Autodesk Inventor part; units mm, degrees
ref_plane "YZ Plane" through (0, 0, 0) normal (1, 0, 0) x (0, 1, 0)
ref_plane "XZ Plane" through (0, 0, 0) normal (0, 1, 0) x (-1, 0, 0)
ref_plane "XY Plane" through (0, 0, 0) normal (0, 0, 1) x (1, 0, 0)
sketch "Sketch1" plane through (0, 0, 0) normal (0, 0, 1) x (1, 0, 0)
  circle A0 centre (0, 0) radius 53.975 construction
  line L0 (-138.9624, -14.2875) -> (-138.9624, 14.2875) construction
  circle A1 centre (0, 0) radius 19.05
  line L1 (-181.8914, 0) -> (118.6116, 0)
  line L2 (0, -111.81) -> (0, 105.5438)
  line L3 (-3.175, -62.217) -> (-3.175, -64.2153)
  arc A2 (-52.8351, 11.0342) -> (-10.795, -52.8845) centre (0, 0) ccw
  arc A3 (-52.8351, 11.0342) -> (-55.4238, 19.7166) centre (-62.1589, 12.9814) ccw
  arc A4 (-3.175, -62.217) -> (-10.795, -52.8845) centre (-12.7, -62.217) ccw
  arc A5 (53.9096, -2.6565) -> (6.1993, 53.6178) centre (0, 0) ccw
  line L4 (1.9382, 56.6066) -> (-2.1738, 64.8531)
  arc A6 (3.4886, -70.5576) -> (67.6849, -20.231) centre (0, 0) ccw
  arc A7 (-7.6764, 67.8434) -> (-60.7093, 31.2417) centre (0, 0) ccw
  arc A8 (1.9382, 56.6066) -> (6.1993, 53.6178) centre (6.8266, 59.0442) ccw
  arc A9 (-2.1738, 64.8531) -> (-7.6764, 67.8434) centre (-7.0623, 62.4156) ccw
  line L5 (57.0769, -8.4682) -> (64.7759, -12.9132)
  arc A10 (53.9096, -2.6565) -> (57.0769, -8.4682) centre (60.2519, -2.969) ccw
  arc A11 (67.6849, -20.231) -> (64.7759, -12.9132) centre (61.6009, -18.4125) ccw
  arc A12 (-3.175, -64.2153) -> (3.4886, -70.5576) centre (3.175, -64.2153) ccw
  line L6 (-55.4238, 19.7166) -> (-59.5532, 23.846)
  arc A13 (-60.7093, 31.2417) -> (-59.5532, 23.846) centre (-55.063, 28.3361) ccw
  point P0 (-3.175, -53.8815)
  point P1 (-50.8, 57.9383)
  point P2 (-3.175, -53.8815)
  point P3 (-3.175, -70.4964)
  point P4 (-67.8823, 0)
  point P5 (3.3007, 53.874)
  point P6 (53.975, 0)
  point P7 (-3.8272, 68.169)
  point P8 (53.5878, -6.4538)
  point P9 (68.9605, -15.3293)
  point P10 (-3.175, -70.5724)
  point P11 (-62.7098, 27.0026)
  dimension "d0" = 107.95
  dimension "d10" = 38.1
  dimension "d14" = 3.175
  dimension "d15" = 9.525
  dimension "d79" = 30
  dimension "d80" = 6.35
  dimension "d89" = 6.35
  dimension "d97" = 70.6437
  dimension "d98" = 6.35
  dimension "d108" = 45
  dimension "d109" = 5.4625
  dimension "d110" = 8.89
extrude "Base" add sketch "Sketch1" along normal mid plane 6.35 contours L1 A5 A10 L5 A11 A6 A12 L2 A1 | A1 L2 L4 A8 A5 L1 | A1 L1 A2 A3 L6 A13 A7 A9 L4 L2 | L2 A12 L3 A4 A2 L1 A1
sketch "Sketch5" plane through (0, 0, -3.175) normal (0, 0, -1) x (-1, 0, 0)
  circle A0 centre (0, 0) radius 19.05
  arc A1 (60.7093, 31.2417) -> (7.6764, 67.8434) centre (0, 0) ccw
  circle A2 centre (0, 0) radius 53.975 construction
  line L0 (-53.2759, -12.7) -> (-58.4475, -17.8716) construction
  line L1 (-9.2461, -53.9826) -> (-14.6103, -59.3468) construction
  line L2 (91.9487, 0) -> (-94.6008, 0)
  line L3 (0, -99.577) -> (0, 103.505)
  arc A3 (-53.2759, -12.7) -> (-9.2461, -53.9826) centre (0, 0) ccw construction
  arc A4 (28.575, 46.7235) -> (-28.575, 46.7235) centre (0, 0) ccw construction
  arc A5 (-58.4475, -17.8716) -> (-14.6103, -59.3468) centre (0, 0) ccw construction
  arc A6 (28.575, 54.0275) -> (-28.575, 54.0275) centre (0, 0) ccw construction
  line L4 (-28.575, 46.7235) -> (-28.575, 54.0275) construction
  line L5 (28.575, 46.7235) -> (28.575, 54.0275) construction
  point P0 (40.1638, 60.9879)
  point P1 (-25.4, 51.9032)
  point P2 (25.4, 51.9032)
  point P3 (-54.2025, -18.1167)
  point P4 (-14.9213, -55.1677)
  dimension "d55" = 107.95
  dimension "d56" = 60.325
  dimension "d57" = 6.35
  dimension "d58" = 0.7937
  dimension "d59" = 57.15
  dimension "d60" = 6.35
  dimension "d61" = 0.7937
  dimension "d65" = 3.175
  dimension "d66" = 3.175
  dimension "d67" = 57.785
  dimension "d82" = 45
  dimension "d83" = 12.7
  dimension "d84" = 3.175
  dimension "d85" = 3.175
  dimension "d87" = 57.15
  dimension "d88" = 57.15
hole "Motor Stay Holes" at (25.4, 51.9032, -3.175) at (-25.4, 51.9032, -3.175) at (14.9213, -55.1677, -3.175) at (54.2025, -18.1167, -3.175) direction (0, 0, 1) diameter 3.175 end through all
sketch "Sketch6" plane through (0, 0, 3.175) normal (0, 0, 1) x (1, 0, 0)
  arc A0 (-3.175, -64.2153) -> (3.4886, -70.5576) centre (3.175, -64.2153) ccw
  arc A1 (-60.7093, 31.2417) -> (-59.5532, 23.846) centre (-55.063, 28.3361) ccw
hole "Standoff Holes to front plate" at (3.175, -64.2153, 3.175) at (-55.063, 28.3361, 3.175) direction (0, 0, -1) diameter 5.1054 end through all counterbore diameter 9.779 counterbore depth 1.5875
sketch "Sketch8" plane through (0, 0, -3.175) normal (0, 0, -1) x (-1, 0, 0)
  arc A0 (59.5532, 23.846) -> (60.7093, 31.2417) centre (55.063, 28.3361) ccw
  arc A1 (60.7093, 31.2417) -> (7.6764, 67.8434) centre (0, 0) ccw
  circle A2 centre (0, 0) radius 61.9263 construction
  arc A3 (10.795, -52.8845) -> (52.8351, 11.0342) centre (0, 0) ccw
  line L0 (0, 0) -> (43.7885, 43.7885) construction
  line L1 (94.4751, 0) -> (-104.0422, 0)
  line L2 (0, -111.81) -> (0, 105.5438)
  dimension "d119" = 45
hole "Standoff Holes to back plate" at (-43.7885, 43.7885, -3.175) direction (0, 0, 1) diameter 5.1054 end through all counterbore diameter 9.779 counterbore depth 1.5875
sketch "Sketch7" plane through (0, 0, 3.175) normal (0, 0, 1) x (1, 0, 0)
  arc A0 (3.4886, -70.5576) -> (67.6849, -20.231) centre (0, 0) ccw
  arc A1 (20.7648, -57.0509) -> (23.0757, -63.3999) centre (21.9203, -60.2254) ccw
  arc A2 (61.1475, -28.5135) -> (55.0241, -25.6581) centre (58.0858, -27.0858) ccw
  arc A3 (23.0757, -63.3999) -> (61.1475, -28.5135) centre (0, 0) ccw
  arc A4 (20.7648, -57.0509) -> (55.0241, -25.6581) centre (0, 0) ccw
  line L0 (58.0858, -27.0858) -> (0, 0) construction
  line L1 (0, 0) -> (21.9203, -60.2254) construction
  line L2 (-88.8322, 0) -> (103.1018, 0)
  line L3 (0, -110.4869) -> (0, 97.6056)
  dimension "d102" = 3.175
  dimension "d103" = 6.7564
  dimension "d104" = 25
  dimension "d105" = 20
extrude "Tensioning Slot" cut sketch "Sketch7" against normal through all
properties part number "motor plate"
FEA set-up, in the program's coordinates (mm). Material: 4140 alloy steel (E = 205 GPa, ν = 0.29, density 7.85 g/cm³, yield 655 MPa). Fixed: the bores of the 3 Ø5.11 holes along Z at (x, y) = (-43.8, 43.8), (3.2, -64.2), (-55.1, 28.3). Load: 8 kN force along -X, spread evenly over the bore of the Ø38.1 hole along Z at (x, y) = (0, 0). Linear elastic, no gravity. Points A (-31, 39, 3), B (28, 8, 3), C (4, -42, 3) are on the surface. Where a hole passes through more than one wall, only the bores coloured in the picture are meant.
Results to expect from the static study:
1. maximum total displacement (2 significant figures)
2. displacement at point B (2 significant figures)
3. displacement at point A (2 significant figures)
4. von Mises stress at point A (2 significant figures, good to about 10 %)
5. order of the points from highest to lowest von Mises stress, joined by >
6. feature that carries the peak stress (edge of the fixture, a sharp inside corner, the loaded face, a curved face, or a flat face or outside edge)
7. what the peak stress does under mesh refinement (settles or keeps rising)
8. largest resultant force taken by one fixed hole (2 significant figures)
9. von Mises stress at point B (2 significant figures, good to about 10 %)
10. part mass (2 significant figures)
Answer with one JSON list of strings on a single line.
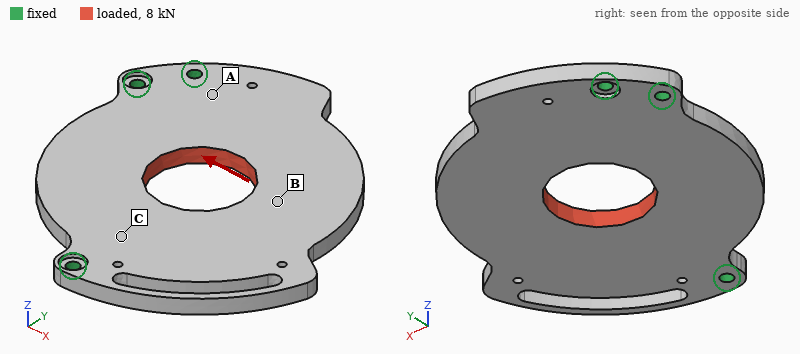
["10 µm", "8.4 µm", "1.9 µm", "27 MPa", "A > B > C", "edge of the fixture", "keeps rising", "3.0 kN", "14 MPa", "500 g"]
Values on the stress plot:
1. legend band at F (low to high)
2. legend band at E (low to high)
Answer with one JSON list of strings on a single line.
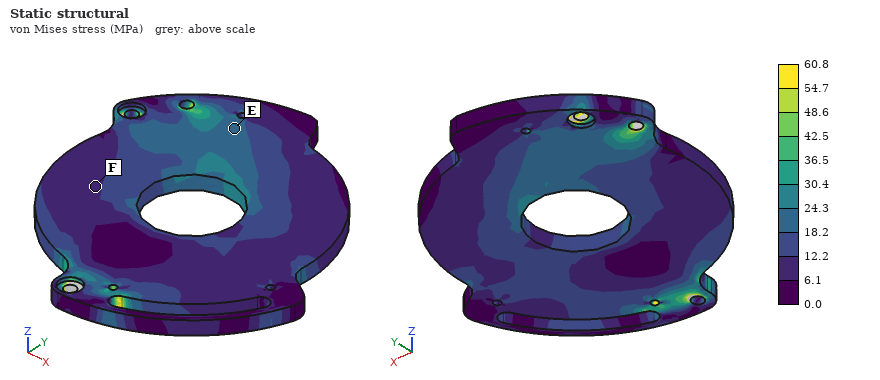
["6.1 to 12.2 MPa", "18.2 to 24.3 MPa"]
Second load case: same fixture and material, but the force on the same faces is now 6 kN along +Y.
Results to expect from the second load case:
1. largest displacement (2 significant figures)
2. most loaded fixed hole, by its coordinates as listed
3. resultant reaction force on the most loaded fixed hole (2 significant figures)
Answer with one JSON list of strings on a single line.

["12 µm", "(3.2, -64.2)", "3.5 kN"]
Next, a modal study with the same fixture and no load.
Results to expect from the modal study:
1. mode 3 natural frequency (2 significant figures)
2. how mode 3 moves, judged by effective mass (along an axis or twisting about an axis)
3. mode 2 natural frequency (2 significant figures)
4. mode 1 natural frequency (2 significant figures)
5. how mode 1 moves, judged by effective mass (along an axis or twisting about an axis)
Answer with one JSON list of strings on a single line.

["2200 Hz", "along Z", "1800 Hz", "670 Hz", "along Z"]
